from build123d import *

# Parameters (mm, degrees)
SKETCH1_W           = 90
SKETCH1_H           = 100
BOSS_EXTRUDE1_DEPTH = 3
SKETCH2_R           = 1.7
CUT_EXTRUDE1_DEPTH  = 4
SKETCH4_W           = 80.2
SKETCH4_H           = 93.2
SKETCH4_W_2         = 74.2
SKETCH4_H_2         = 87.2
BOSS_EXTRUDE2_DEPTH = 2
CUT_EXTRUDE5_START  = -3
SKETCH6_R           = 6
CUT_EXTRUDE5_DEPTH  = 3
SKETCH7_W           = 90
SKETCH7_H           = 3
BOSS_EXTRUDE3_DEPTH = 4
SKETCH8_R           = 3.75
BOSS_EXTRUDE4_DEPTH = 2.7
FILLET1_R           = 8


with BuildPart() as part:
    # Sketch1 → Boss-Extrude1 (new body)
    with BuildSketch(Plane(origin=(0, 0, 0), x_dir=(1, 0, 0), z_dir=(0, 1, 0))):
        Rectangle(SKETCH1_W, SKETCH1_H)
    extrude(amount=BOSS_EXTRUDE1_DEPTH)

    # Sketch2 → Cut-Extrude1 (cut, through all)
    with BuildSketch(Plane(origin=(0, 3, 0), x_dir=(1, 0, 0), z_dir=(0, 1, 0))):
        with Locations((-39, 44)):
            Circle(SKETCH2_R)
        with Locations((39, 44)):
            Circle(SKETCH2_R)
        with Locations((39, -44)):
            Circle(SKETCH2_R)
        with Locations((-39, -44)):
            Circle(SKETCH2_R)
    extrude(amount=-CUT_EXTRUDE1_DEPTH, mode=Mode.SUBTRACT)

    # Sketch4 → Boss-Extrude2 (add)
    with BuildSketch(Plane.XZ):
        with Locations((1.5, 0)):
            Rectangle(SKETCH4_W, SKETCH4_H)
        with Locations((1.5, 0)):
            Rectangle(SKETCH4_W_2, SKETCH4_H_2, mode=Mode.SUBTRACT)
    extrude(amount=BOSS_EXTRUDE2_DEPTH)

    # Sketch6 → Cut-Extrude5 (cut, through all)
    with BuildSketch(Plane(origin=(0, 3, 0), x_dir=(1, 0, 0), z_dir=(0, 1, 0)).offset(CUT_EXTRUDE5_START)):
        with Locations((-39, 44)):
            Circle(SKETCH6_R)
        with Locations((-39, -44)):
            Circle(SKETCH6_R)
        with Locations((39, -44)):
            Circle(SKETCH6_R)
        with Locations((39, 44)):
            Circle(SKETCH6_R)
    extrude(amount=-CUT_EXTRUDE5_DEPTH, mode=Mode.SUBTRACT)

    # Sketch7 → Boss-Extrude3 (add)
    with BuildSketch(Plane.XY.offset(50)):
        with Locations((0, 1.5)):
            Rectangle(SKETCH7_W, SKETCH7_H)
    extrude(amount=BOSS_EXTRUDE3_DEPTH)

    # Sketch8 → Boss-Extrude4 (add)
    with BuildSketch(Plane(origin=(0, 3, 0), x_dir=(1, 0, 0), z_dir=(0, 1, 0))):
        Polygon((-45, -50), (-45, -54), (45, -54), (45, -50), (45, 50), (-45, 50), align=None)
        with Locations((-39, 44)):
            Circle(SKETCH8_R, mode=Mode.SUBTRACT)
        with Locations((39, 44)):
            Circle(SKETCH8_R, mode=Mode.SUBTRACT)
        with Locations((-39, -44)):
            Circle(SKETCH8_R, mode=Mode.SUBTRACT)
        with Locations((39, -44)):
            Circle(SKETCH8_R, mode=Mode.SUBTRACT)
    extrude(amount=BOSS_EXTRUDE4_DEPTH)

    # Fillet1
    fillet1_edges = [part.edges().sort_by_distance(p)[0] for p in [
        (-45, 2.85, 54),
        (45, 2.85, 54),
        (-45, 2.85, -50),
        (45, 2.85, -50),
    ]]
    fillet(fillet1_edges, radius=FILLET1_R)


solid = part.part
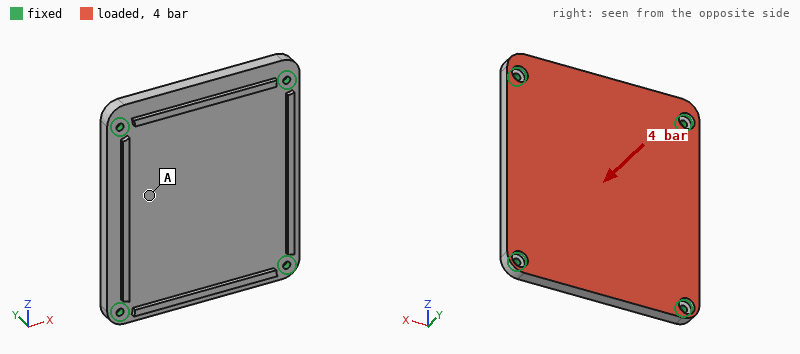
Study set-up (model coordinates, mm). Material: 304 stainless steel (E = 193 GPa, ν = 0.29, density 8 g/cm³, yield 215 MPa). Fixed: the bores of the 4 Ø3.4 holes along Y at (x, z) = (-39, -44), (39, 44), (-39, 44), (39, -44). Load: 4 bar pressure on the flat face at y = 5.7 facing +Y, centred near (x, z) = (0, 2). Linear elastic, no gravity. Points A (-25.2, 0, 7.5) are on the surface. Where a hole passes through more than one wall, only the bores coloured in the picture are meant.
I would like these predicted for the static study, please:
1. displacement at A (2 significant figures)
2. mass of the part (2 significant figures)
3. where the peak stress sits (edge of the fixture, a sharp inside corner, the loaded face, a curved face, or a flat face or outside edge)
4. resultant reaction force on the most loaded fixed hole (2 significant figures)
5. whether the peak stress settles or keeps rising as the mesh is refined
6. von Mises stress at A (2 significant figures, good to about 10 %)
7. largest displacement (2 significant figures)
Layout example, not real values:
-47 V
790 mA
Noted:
57 µm
430 g
edge of the fixture
1.5 kN
keeps rising
29 MPa
69 µm
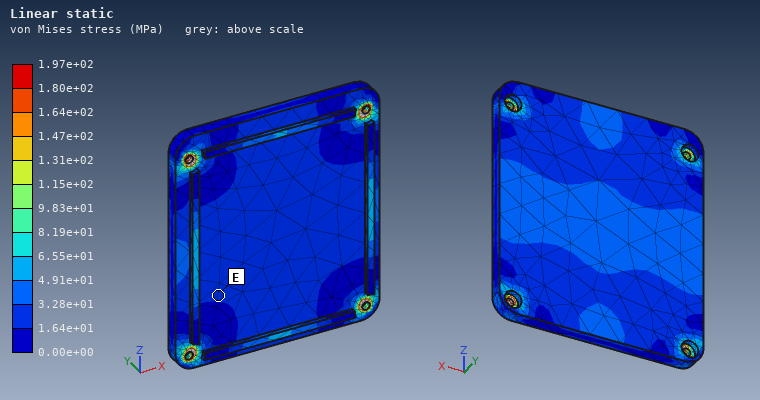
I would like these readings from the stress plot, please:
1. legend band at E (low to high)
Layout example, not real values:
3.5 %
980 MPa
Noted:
1.64e+01 to 3.28e+01 MPa
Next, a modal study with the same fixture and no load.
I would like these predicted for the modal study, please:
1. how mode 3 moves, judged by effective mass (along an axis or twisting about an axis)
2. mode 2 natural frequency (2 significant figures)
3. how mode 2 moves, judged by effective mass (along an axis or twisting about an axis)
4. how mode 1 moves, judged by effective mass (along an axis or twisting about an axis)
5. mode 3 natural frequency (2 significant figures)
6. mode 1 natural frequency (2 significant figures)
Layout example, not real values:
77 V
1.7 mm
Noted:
twisting about X
3600 Hz
twisting about Z
along Y
3900 Hz
2100 Hz
